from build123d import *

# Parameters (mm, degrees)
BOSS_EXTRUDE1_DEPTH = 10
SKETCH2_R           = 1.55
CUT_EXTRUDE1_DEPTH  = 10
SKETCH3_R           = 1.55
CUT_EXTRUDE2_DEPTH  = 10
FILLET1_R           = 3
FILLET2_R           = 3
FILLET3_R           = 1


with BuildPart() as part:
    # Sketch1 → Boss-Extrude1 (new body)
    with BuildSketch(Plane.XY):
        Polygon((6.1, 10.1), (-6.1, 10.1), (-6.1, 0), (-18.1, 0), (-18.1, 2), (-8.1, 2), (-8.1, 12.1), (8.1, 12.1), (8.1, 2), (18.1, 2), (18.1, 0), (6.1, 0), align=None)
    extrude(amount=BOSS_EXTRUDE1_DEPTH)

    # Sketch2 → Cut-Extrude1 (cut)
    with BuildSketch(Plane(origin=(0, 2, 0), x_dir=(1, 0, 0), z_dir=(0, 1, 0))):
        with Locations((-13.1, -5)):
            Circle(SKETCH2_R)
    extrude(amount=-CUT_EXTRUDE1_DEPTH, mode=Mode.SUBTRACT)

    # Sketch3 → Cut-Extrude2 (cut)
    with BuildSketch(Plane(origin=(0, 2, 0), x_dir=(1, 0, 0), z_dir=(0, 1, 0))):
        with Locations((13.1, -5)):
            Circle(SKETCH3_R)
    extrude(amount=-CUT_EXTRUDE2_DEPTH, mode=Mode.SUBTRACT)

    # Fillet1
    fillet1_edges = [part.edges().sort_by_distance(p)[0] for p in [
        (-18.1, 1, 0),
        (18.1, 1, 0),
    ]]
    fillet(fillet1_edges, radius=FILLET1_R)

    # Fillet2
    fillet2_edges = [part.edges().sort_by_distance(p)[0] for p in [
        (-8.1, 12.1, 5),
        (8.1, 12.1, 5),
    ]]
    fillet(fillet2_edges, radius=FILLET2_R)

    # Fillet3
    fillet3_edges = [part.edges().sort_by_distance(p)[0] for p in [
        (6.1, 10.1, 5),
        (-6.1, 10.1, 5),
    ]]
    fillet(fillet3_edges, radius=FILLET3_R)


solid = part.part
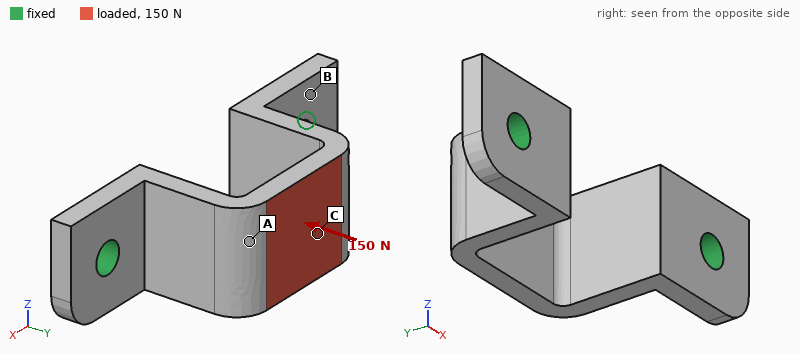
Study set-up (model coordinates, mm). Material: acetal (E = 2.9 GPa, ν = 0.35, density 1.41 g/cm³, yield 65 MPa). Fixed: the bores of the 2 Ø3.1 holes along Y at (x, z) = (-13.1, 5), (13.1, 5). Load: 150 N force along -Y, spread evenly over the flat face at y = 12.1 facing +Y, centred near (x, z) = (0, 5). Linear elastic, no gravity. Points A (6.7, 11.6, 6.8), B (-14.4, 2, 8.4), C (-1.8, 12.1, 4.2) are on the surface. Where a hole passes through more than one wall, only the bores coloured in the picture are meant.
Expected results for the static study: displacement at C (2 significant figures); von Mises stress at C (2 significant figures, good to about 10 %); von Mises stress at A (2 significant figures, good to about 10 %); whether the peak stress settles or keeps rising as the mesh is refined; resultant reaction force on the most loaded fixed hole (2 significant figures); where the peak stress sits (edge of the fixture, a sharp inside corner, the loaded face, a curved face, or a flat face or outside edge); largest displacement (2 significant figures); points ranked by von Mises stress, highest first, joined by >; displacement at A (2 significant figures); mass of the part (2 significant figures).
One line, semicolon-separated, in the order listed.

0.19 mm; 17 MPa; 8.9 MPa; keeps rising; 84 N; edge of the fixture; 0.22 mm; C > A > B; 0.097 mm; 1.5 g
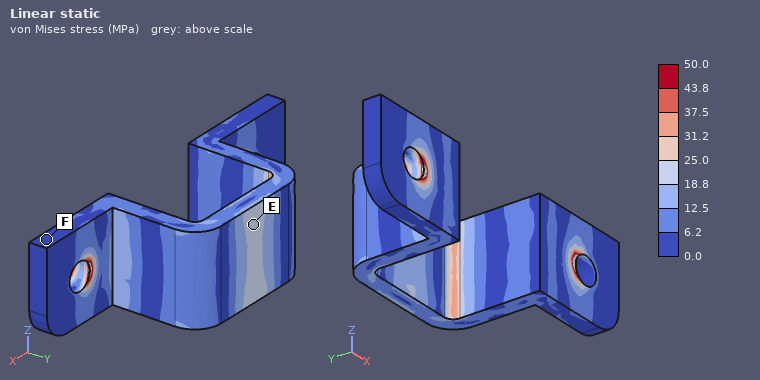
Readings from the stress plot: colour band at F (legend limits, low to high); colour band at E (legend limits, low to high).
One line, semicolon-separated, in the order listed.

0.0 to 6.2 MPa; 18.8 to 25.0 MPa
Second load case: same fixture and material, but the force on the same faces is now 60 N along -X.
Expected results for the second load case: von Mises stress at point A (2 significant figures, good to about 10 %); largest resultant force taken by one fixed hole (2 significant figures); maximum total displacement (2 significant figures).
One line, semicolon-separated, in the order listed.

11 MPa; 40 N; 0.24 mm
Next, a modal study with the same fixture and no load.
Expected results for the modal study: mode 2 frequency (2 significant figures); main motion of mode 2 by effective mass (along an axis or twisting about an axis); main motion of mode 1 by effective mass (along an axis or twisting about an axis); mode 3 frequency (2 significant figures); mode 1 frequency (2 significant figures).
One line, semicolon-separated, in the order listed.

3200 Hz; along X; along Z; 4500 Hz; 2300 Hz
